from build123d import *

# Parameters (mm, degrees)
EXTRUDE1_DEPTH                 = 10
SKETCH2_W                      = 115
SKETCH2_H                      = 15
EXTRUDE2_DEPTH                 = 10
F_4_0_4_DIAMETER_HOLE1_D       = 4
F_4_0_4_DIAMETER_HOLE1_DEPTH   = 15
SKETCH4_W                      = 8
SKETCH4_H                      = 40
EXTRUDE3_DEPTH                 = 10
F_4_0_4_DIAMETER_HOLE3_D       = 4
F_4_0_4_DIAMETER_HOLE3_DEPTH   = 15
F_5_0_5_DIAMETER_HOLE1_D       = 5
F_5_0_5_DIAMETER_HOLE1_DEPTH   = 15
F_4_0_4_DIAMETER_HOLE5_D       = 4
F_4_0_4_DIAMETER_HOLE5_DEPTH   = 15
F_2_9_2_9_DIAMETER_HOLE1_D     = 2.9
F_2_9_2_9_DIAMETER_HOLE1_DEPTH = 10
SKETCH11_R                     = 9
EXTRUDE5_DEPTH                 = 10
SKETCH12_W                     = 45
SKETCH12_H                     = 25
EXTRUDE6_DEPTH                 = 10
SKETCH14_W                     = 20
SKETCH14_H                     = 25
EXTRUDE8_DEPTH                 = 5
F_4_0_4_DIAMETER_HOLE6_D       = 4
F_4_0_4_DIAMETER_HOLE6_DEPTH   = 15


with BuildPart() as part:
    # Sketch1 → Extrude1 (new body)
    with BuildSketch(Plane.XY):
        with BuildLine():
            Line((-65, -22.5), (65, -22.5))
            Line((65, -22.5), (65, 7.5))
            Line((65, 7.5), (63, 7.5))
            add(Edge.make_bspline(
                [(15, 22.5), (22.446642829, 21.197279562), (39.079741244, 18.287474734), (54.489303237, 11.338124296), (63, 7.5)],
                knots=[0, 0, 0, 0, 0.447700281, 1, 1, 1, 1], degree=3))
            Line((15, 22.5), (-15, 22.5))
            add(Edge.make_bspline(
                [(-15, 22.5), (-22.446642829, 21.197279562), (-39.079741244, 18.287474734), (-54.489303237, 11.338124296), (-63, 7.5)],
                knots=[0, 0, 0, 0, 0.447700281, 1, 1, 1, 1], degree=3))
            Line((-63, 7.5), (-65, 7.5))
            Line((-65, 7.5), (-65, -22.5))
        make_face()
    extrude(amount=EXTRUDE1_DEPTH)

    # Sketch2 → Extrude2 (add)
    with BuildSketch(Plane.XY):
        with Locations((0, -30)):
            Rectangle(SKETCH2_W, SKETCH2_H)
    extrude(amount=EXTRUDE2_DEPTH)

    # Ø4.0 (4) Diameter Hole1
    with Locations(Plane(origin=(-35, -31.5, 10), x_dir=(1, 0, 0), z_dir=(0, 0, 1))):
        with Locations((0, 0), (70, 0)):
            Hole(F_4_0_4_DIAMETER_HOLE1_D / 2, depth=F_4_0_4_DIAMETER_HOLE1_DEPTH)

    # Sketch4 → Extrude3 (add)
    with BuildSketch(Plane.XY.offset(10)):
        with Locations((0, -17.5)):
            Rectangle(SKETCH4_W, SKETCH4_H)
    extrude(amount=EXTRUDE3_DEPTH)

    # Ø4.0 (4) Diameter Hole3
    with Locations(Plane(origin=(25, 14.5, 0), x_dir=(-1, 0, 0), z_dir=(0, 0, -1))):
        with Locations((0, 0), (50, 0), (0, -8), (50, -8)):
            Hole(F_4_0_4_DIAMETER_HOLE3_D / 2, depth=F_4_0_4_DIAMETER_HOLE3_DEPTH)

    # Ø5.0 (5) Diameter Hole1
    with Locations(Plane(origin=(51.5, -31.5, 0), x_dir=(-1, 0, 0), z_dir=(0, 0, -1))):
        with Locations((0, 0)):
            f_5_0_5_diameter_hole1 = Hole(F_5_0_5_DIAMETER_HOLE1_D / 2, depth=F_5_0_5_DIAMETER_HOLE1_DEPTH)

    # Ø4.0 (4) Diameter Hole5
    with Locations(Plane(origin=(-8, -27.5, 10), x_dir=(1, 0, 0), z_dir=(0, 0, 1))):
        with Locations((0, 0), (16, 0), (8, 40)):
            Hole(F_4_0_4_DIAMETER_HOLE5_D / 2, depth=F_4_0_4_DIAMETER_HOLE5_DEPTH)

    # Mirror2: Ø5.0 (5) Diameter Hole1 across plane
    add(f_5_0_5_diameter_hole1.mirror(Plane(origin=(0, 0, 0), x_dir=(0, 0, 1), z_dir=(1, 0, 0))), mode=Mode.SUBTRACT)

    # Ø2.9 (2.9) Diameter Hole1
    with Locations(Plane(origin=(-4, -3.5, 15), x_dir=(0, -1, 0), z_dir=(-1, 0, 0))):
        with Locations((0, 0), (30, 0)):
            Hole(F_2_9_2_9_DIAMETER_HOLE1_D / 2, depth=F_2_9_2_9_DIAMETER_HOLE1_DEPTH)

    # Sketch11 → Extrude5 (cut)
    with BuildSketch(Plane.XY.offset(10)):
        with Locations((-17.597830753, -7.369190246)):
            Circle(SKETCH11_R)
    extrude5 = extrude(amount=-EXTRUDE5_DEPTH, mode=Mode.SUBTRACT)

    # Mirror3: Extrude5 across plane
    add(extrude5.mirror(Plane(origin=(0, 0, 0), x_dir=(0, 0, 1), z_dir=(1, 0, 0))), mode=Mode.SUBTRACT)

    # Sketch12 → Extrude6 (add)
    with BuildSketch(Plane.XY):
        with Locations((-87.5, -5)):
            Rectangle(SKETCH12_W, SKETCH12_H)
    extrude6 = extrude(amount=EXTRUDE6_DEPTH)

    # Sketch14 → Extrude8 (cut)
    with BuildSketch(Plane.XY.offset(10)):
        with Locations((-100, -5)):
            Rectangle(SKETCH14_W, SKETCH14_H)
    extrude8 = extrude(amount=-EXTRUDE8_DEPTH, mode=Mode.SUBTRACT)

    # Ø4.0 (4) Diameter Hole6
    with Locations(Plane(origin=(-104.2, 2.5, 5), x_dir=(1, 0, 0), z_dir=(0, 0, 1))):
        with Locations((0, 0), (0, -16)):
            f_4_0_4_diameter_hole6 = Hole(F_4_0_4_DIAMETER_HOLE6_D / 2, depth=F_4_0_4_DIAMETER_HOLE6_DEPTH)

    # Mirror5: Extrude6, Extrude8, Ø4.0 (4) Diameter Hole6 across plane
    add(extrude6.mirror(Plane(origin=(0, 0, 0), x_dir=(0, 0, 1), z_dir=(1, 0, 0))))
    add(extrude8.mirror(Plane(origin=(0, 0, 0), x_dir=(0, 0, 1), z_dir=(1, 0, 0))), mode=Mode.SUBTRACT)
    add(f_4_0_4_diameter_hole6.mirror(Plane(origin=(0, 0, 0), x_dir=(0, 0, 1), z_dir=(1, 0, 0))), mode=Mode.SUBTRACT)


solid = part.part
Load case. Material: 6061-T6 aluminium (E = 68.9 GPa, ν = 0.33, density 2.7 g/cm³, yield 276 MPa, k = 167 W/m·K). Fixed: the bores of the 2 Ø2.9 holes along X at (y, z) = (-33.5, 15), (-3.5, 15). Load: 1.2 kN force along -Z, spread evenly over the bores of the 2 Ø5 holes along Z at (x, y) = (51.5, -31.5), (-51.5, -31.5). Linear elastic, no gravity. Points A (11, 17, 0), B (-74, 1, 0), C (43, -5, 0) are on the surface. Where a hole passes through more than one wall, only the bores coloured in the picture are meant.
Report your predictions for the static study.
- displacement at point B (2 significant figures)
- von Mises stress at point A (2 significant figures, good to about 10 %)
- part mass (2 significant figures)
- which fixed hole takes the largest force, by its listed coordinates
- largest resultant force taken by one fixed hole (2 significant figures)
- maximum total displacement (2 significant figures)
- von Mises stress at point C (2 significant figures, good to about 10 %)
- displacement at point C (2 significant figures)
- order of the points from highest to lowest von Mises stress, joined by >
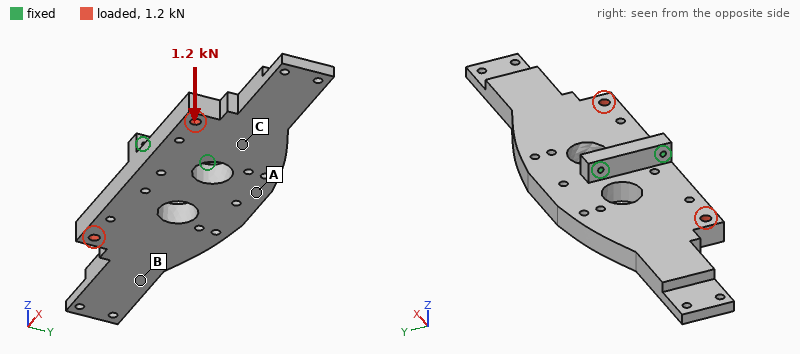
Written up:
0.16 mm
20 MPa
220 g
(-33.5, 15)
1.2 kN
0.29 mm
12 MPa
0.078 mm
A > C > B
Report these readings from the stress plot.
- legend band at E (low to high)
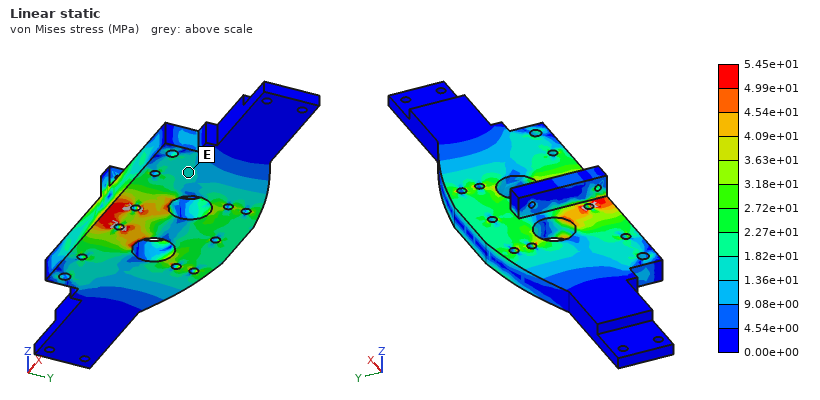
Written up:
1.36e+01 to 1.82e+01 MPa
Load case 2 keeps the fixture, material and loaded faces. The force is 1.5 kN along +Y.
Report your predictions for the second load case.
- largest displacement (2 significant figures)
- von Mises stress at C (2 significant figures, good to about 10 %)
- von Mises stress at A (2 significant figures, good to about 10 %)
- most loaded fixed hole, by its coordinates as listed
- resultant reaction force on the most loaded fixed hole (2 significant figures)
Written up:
15 µm
3.5 MPa
5.2 MPa
(-3.5, 15)
930 N
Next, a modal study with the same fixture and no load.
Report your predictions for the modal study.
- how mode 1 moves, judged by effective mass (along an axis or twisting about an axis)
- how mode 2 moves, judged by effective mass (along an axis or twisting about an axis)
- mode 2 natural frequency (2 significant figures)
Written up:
twisting about Y
along Z
1000 Hz
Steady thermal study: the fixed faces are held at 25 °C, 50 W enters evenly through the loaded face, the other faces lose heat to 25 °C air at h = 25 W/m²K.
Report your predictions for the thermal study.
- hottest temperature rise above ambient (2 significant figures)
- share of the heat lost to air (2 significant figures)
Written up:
33 K
21 %
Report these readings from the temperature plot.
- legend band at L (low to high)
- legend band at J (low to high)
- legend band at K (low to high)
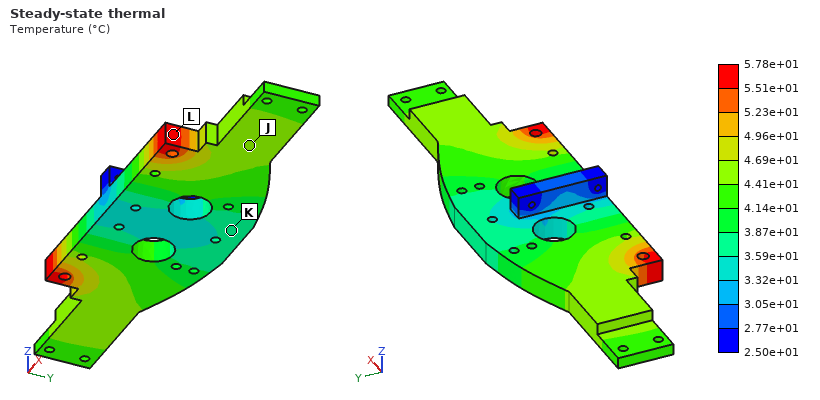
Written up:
5.51e+01 to 5.78e+01 °C
4.41e+01 to 4.69e+01 °C
3.59e+01 to 3.87e+01 °C
